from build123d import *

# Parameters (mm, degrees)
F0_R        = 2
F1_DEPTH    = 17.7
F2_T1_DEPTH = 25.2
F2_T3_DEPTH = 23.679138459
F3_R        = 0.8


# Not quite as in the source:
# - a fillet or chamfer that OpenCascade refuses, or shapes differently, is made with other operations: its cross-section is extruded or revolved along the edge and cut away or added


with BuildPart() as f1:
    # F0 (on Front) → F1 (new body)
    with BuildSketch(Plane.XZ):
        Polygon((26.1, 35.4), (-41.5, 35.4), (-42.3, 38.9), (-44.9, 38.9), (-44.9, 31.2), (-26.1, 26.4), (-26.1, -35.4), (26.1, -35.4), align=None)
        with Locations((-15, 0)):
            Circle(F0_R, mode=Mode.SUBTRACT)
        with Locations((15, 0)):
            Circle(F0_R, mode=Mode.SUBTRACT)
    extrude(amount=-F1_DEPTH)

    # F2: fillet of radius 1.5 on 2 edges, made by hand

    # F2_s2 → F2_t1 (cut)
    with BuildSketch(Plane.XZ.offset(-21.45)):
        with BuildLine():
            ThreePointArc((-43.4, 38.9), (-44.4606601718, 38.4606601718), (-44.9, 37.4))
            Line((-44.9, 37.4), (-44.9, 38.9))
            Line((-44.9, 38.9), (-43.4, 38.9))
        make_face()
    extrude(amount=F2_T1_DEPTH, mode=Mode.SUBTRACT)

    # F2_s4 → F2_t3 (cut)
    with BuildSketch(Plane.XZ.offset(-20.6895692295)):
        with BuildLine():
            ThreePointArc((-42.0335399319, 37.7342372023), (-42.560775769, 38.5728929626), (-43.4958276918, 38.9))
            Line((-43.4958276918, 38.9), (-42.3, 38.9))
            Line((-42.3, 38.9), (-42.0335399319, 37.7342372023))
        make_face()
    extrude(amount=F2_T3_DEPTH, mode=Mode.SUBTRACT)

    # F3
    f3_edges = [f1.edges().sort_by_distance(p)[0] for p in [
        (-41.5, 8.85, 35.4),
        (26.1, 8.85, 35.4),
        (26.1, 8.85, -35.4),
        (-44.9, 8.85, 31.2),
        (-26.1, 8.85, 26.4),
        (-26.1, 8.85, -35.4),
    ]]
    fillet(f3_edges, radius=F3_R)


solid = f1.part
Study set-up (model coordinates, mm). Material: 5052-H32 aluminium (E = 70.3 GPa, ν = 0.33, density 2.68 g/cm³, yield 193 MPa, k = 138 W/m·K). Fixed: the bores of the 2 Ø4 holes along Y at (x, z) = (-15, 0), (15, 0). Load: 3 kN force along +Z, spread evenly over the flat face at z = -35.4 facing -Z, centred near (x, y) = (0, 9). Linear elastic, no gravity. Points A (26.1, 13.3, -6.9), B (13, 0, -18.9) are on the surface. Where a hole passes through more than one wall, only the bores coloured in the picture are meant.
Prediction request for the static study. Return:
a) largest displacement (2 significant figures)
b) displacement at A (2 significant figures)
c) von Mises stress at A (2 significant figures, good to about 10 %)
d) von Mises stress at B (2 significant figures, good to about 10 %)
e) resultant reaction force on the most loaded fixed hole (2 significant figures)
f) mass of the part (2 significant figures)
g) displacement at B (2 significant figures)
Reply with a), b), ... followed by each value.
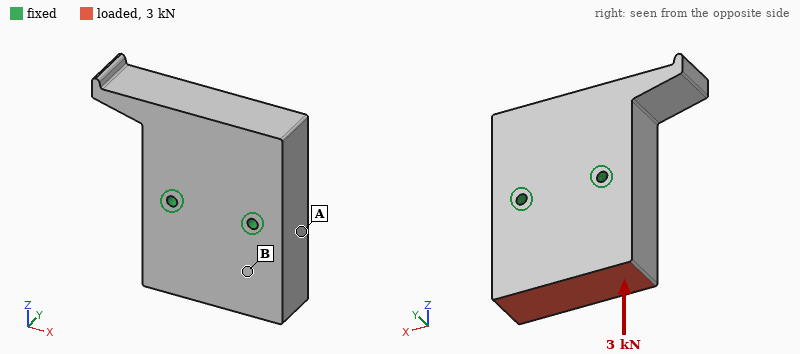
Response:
a) 2.0 µm
b) 0.84 µm
c) 1.8 MPa
d) 3.6 MPa
e) 1.5 kN
f) 180 g
g) 1.2 µm
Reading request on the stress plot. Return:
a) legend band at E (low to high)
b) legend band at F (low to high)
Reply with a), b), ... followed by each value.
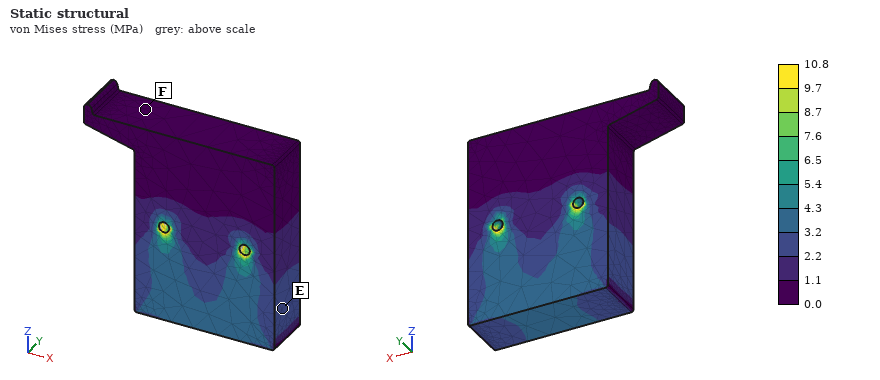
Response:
a) 2.2 to 3.2 MPa
b) 0.0 to 1.1 MPa
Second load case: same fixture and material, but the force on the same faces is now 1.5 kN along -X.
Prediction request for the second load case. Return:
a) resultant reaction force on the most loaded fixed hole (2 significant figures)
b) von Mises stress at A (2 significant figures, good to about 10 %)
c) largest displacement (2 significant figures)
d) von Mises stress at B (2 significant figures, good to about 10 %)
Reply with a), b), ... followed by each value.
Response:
a) 1.8 kN
b) 3.8 MPa
c) 6.2 µm
d) 3.5 MPa
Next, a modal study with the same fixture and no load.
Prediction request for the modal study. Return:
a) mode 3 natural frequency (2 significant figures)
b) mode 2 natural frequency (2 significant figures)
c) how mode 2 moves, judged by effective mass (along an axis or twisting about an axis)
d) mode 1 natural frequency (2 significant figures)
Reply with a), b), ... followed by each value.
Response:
a) 11 kHz
b) 9200 Hz
c) along Y
d) 6800 Hz
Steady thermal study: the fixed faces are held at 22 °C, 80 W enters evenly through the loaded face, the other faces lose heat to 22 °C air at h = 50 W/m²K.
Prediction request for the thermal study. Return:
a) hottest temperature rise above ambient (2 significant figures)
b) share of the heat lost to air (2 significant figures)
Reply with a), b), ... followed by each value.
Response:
a) 24 K
b) 4.7 %
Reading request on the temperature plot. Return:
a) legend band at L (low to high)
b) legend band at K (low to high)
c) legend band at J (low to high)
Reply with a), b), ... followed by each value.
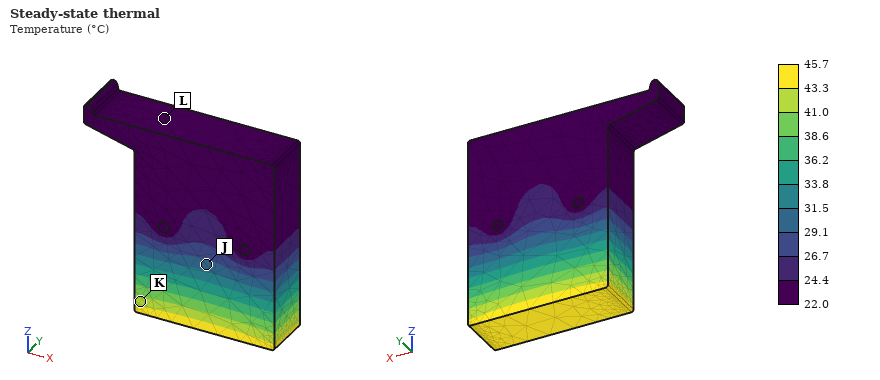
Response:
a) 22.0 to 24.4 °C
b) 41.0 to 43.3 °C
c) 29.1 to 31.5 °C
